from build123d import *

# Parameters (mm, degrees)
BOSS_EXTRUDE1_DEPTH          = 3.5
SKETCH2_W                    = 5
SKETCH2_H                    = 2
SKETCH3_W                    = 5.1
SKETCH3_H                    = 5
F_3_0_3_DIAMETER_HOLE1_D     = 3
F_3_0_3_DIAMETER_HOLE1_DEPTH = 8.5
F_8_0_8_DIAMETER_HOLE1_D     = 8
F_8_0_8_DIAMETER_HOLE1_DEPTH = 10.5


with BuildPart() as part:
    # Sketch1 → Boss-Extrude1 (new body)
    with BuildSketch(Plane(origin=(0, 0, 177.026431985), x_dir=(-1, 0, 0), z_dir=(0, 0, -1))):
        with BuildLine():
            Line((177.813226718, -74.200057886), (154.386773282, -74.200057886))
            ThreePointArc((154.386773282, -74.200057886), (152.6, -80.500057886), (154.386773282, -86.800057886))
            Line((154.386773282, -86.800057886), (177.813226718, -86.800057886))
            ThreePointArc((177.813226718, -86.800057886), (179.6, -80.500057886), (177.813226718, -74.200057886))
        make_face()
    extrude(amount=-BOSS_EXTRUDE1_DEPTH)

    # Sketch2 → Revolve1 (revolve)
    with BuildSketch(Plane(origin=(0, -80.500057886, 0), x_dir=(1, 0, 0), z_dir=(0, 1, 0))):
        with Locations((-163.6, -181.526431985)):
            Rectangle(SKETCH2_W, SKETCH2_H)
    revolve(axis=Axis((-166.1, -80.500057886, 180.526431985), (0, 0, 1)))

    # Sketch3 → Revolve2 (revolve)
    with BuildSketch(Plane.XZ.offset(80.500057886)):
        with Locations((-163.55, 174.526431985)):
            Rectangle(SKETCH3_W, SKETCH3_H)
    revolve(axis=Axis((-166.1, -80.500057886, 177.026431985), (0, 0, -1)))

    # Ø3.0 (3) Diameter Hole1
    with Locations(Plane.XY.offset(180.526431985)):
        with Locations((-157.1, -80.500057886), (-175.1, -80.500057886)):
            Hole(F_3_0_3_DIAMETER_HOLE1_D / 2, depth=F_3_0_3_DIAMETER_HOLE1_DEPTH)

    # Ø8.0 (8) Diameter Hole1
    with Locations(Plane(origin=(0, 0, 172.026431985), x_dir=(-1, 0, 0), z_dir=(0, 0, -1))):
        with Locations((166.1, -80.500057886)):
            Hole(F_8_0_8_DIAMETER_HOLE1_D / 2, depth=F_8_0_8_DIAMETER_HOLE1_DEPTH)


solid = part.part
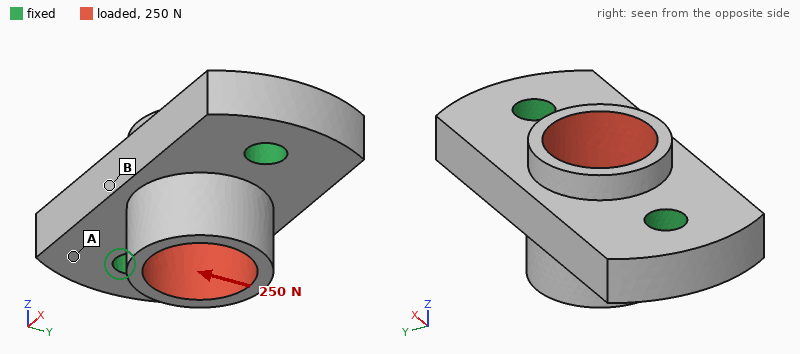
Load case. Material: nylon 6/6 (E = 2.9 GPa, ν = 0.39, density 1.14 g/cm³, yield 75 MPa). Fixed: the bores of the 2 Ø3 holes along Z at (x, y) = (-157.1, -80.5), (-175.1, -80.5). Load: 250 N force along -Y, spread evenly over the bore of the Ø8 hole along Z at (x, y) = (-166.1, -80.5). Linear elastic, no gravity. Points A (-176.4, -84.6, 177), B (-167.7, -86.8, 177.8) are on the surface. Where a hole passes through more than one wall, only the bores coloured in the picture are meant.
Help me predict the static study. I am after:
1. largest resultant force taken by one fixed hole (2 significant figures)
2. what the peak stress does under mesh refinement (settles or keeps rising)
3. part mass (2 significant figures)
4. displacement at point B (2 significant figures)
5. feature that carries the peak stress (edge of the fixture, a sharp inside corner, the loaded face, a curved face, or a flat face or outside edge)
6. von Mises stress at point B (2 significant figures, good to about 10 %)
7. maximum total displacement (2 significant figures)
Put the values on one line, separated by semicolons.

130 N; keeps rising; 1.3 g; 50 µm; edge of the fixture; 6.8 MPa; 98 µm
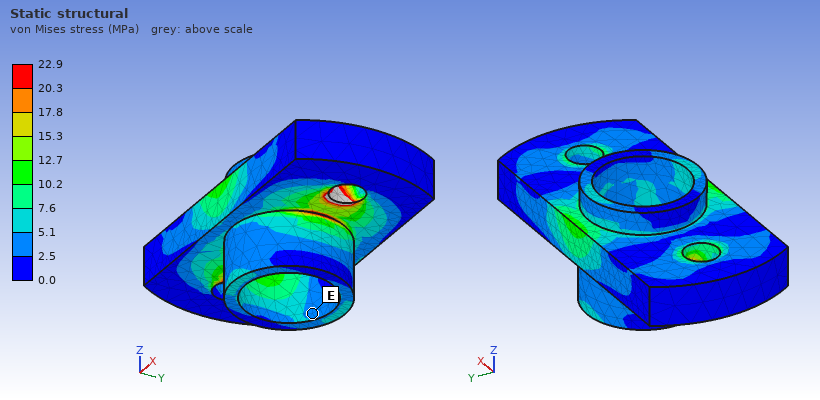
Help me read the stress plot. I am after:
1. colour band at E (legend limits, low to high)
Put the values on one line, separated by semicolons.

2.5 to 5.1 MPa
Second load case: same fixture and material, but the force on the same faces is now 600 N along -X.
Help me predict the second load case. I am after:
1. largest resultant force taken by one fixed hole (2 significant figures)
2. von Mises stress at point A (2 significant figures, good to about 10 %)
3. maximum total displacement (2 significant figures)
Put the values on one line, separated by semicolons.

310 N; 2.8 MPa; 0.10 mm
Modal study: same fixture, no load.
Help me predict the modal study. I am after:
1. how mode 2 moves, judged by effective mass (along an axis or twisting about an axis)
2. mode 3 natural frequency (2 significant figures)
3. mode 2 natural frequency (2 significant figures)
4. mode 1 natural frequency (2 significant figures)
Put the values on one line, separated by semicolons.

along Z; 18 kHz; 13 kHz; 10 kHz
